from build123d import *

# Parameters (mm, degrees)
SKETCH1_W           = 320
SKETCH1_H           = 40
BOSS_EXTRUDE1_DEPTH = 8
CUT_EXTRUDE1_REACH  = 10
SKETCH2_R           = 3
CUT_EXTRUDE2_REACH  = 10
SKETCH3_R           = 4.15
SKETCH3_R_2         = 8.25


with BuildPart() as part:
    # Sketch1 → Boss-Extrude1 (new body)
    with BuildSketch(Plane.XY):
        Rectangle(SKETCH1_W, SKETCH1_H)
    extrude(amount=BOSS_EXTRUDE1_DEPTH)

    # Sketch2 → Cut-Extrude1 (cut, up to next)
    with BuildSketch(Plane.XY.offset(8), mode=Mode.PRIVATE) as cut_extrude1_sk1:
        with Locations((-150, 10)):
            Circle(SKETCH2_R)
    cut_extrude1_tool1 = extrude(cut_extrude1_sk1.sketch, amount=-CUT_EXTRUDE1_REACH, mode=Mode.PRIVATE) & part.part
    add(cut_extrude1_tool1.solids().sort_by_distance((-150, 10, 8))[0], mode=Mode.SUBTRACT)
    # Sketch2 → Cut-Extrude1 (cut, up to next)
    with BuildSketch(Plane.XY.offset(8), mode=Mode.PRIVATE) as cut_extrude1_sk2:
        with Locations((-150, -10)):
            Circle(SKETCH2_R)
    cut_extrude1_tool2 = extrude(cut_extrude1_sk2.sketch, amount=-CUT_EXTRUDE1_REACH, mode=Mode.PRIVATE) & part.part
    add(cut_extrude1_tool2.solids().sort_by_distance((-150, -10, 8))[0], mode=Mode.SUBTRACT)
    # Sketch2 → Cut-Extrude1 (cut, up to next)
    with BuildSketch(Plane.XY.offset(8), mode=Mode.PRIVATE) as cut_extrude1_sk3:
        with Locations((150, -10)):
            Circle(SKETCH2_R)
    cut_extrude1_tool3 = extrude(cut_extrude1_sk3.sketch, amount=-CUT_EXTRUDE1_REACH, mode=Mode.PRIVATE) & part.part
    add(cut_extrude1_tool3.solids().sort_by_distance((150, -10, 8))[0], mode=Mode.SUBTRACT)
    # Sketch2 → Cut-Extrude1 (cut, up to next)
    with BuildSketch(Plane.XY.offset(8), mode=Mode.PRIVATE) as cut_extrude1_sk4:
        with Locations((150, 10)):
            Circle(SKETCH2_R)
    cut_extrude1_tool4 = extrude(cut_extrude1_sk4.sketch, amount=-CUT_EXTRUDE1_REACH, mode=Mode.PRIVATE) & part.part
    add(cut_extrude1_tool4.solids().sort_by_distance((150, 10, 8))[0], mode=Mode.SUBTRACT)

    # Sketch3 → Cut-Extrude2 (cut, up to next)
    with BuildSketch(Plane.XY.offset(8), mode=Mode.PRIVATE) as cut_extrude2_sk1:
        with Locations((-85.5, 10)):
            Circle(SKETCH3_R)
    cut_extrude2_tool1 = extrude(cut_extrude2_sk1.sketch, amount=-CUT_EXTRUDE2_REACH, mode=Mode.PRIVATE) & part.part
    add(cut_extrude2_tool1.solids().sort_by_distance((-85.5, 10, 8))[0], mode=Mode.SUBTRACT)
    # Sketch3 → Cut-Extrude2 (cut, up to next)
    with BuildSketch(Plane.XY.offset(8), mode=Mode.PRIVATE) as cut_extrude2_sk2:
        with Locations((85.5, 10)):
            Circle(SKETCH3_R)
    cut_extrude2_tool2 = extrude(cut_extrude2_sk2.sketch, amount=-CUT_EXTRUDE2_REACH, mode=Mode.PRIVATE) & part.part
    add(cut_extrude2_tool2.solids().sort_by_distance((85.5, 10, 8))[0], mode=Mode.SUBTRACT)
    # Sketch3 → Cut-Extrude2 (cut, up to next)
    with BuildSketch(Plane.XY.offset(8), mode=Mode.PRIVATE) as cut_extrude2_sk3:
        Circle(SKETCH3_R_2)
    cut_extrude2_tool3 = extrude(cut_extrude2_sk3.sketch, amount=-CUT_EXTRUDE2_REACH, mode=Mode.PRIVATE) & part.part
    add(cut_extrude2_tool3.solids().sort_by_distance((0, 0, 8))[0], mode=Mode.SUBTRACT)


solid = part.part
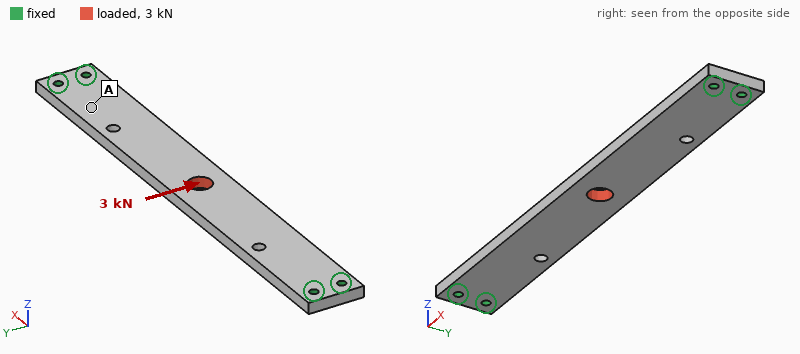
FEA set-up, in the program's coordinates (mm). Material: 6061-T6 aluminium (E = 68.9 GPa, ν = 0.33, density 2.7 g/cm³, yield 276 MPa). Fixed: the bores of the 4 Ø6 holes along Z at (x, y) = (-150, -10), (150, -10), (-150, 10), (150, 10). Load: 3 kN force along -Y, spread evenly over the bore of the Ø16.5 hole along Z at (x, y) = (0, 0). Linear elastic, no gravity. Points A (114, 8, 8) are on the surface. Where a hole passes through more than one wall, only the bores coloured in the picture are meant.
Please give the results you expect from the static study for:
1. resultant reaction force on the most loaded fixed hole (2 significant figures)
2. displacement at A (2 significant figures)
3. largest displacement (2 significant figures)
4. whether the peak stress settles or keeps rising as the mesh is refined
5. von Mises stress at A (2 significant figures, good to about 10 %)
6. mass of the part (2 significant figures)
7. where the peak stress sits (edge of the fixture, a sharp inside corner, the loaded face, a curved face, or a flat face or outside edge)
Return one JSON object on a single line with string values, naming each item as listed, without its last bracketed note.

{"resultant reaction force on the most loaded fixed hole": "4.6 kN", "displacement at A": "0.034 mm", "largest displacement": "0.19 mm", "whether the peak stress settles or keeps rising as the mesh is refined": "keeps rising", "von Mises stress at A": "15 MPa", "mass of the part": "270 g", "where the peak stress sits": "edge of the fixture"}
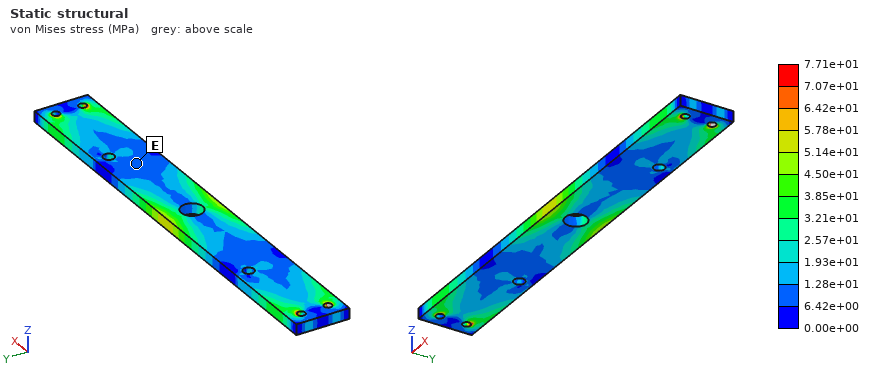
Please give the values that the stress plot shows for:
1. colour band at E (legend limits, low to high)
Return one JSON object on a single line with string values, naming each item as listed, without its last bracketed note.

{"colour band at E": "6.42e+00 to 1.28e+01 MPa"}
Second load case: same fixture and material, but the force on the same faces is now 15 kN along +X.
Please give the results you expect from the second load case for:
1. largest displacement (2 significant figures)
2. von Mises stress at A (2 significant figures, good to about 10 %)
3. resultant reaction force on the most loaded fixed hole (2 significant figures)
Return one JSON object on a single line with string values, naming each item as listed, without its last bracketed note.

{"largest displacement": "55 µm", "von Mises stress at A": "23 MPa", "resultant reaction force on the most loaded fixed hole": "3.9 kN"}
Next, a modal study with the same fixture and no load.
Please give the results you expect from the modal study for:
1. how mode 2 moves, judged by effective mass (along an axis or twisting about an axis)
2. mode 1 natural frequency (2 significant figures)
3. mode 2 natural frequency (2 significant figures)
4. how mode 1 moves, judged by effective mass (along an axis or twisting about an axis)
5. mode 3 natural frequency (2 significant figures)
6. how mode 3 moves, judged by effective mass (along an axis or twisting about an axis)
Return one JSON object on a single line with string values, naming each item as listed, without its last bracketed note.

{"how mode 2 moves, judged by effective mass": "twisting about Y", "mode 1 natural frequency": "470 Hz", "mode 2 natural frequency": "1300 Hz", "how mode 1 moves, judged by effective mass": "along Z", "mode 3 natural frequency": "2000 Hz", "how mode 3 moves, judged by effective mass": "twisting about X"}
